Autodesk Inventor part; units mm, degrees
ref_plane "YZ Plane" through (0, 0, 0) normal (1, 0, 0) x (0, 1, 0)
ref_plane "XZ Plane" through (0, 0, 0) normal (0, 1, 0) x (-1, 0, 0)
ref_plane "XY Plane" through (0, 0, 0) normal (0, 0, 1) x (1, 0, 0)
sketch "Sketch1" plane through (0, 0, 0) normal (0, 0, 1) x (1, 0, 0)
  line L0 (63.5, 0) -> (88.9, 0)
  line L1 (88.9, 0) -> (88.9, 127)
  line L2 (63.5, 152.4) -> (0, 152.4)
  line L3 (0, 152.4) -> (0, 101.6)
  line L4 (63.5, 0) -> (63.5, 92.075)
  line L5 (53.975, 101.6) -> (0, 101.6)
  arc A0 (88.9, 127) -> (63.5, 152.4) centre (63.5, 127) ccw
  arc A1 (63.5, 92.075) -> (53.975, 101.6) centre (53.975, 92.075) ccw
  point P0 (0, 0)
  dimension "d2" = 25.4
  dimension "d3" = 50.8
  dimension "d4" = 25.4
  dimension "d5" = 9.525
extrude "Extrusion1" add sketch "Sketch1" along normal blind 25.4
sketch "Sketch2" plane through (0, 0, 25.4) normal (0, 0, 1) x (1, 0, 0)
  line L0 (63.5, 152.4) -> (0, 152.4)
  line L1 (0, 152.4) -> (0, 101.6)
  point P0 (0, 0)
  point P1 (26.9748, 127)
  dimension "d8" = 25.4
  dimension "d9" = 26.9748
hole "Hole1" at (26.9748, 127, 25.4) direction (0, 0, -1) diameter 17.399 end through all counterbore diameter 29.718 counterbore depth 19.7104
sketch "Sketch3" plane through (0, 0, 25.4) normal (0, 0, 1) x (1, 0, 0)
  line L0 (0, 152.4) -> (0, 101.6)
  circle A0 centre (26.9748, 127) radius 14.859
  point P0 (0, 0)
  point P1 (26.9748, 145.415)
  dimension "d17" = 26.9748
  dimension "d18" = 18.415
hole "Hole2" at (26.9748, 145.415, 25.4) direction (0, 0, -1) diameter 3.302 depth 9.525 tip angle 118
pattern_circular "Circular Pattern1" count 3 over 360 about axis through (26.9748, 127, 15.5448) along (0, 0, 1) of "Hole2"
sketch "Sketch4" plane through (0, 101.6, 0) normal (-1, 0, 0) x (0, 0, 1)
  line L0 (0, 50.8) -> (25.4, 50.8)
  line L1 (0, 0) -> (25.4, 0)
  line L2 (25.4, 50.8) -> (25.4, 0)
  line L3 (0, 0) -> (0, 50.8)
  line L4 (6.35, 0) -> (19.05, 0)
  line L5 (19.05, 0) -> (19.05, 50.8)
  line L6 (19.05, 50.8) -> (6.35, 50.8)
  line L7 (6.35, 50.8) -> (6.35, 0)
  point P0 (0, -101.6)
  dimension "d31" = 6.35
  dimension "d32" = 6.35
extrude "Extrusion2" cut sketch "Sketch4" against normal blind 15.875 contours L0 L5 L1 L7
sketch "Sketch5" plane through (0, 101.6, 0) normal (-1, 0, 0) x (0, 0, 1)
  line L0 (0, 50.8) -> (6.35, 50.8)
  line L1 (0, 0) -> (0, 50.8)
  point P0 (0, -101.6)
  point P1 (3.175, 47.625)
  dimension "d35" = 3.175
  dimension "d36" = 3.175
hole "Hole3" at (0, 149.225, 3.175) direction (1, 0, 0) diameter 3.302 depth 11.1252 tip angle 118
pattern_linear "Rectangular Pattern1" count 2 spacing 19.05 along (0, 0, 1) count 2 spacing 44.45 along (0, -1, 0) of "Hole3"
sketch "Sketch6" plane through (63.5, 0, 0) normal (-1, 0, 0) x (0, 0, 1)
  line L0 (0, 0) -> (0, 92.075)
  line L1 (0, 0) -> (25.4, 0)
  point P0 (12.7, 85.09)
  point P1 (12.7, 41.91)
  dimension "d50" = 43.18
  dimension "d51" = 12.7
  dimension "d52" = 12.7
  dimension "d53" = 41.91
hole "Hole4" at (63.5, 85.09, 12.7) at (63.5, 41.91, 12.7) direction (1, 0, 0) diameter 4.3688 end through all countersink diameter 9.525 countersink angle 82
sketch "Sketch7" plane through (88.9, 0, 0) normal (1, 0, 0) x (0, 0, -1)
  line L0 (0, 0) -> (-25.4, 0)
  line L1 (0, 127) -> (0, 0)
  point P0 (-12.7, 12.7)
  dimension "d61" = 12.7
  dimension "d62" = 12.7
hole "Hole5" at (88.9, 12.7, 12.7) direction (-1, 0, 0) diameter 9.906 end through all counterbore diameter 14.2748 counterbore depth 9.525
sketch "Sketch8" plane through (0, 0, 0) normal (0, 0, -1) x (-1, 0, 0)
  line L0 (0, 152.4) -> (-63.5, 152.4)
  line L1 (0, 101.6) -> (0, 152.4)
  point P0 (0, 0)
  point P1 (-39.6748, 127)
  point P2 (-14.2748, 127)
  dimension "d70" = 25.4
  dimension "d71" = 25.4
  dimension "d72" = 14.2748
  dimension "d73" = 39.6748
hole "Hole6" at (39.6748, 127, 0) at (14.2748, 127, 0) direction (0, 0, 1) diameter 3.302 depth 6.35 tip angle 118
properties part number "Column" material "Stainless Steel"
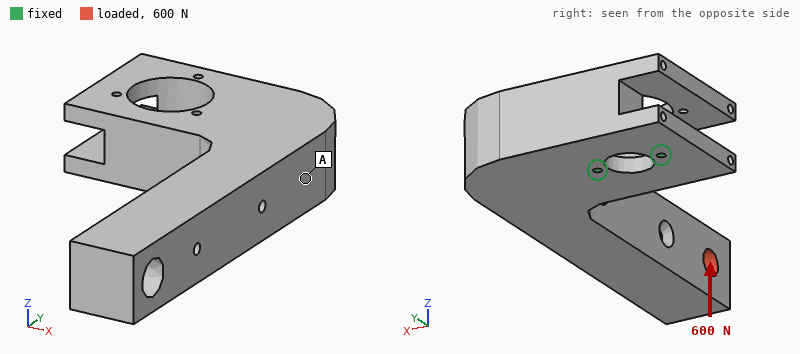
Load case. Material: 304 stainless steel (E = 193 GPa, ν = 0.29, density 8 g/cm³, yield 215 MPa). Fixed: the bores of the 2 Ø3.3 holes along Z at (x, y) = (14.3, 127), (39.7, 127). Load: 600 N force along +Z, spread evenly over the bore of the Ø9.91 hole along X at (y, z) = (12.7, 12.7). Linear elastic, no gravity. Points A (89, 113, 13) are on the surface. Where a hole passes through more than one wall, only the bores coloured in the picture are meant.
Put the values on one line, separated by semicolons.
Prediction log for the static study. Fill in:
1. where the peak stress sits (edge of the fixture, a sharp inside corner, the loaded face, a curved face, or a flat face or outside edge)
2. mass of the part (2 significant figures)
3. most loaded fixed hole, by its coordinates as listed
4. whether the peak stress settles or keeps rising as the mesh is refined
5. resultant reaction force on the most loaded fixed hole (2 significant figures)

edge of the fixture; 1.2 kg; (39.7, 127); keeps rising; 1.2 kN
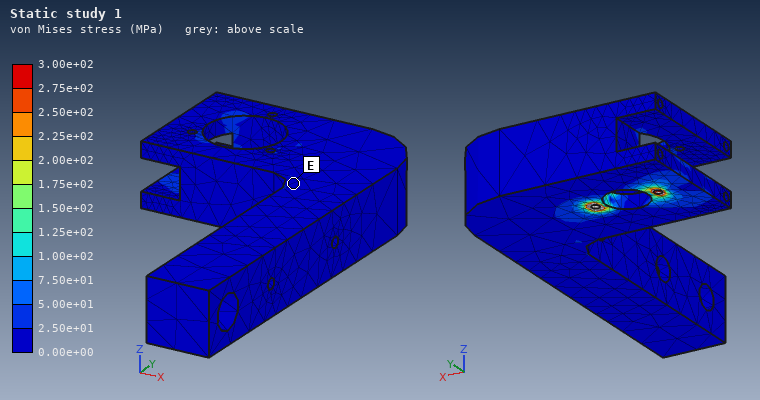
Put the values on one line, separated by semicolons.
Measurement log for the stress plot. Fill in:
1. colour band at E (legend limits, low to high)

0.00e+00 to 2.50e+01 MPa
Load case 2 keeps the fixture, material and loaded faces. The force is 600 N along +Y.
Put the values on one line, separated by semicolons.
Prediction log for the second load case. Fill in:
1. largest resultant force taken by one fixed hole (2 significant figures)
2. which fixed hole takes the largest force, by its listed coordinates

1.2 kN; (39.7, 127)
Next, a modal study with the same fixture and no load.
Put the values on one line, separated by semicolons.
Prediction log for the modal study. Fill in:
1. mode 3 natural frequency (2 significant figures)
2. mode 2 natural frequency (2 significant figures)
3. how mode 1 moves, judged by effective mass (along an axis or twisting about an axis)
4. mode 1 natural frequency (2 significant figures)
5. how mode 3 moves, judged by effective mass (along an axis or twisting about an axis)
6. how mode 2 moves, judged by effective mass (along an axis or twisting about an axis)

1800 Hz; 960 Hz; along Z; 400 Hz; along Z; along X
